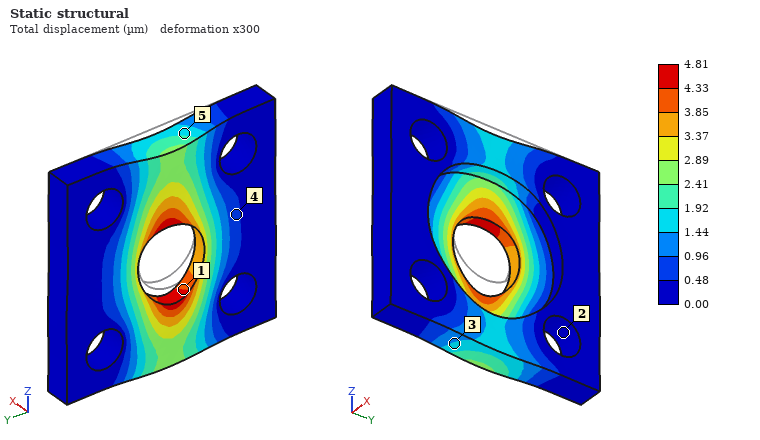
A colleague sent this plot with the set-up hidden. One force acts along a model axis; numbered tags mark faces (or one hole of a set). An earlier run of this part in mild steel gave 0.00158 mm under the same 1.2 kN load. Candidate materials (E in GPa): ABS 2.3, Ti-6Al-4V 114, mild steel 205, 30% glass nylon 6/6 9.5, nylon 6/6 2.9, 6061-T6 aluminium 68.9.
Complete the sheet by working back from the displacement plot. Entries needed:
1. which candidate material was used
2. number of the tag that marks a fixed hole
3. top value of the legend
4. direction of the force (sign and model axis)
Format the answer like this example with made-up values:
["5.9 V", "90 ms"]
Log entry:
["6061-T6 aluminium", "2", "4.81 µm", "-Z"]
